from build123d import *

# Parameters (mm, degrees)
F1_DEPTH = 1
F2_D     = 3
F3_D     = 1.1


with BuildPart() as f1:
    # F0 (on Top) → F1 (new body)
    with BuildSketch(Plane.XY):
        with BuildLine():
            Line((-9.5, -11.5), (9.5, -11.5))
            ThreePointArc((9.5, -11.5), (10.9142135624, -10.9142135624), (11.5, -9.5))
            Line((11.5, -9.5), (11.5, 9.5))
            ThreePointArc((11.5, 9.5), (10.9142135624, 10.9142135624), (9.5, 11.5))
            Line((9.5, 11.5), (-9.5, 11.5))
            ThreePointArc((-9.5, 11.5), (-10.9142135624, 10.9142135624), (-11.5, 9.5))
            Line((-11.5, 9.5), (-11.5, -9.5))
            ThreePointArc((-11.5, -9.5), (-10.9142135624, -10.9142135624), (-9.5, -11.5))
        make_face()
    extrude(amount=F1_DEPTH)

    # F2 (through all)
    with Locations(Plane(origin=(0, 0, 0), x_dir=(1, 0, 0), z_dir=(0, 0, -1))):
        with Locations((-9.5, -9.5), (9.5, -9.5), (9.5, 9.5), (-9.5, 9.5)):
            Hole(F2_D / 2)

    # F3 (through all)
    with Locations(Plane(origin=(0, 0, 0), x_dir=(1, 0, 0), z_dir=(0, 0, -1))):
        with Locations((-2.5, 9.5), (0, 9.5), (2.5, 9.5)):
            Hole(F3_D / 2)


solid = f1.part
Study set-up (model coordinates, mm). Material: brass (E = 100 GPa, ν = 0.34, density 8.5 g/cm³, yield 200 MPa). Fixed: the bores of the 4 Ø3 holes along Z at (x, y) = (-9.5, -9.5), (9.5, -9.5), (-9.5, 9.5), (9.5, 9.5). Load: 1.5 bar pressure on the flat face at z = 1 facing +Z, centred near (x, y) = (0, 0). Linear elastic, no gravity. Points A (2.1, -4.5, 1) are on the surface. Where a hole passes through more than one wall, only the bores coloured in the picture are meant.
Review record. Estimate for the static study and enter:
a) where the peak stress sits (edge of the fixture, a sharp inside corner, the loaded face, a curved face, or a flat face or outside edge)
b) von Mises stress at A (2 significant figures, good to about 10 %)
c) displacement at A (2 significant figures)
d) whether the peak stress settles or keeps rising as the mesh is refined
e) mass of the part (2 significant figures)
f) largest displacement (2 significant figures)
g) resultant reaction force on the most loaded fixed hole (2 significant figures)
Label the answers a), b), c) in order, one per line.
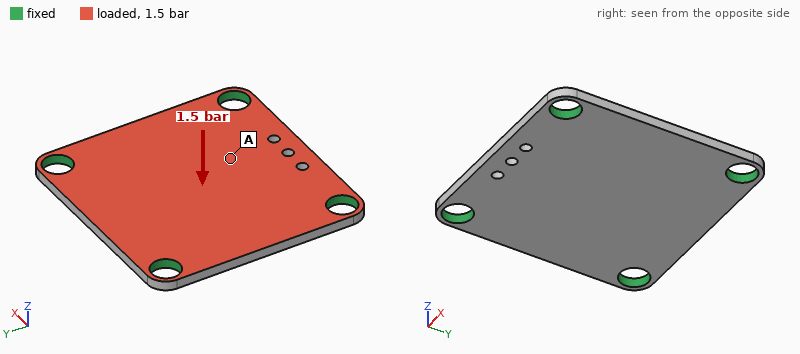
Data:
a) edge of the fixture
b) 11 MPa
c) 8.0 µm
d) keeps rising
e) 4.2 g
f) 10 µm
g) 19 N
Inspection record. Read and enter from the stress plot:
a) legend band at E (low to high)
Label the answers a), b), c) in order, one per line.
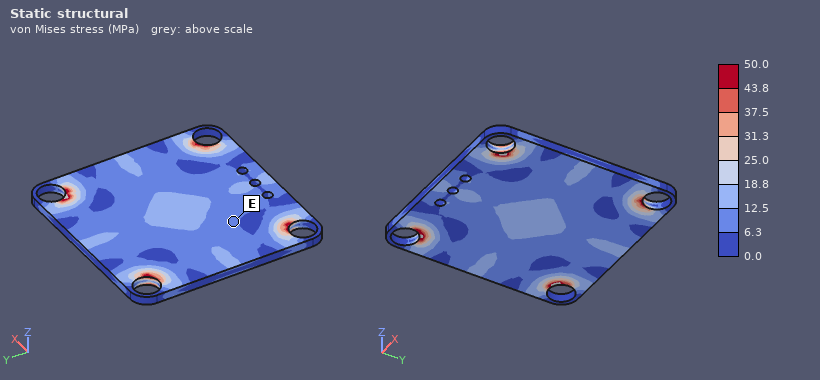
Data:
a) 6.3 to 12.5 MPa
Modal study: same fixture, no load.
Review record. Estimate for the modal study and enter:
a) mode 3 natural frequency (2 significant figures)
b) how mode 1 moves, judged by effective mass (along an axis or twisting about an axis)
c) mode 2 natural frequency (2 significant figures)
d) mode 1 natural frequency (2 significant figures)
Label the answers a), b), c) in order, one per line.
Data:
a) 14 kHz
b) along Z
c) 13 kHz
d) 8200 Hz
